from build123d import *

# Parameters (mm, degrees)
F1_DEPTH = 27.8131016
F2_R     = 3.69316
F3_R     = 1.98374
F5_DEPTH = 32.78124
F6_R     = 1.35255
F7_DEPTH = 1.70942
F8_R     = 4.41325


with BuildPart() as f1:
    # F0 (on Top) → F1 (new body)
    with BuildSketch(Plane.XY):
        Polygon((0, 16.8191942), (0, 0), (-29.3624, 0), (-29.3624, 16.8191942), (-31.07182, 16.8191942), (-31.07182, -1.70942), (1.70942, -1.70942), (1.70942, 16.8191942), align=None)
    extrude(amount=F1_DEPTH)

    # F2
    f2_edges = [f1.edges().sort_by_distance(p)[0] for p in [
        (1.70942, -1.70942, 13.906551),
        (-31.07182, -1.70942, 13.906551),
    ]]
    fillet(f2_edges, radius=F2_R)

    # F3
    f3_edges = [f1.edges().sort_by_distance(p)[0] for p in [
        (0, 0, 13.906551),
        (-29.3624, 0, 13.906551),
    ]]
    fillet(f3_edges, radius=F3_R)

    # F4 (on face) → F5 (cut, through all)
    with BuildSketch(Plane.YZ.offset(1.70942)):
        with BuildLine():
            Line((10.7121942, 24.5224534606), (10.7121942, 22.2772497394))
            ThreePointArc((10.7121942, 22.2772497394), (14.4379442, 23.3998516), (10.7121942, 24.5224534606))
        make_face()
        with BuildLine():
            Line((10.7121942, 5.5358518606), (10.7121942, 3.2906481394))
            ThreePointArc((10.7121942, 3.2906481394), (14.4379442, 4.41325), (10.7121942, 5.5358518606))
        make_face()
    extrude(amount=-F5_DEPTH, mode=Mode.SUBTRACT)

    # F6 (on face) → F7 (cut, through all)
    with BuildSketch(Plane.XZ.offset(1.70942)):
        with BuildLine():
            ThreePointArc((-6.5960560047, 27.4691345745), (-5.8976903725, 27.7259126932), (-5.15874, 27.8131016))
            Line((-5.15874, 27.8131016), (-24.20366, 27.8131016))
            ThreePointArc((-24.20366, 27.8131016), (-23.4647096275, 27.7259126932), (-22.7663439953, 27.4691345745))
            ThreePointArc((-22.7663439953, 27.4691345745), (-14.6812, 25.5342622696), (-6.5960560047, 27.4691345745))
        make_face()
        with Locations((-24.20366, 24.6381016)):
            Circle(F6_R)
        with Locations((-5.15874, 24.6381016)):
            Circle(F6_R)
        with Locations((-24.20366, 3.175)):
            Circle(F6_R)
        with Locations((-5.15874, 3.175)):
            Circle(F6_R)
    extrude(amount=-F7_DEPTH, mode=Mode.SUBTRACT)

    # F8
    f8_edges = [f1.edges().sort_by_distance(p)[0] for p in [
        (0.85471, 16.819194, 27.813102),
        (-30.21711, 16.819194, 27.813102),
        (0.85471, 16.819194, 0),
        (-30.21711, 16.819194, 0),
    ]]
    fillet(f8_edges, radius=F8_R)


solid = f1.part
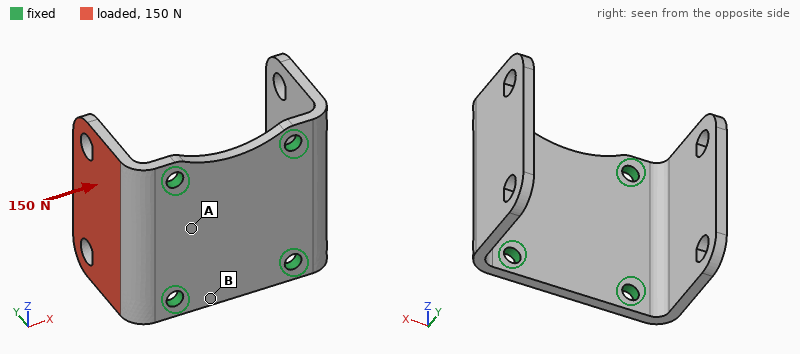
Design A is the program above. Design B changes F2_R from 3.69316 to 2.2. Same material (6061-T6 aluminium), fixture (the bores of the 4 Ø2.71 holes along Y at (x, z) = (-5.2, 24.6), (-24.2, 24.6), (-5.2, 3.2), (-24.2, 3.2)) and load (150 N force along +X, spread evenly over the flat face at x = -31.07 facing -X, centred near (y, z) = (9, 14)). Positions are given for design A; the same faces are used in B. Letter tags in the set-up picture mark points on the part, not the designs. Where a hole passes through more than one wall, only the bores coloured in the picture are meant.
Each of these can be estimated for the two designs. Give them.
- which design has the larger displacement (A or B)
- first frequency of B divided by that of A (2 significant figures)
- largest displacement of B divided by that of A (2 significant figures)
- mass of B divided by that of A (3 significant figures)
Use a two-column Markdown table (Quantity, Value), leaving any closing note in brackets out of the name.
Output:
| Quantity | Value |
|---|---|
| which design has the larger displacement | A |
| first frequency of B divided by that of A | 1.1 |
| largest displacement of B divided by that of A | 0.81 |
| mass of B divided by that of A | 1.04 |
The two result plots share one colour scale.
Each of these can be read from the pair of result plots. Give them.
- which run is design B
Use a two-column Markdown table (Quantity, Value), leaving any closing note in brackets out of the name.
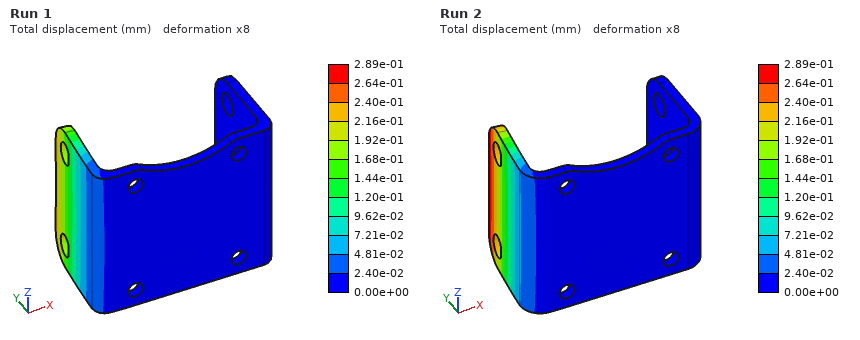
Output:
| Quantity | Value |
|---|---|
| which run is design B | Run 1 |
